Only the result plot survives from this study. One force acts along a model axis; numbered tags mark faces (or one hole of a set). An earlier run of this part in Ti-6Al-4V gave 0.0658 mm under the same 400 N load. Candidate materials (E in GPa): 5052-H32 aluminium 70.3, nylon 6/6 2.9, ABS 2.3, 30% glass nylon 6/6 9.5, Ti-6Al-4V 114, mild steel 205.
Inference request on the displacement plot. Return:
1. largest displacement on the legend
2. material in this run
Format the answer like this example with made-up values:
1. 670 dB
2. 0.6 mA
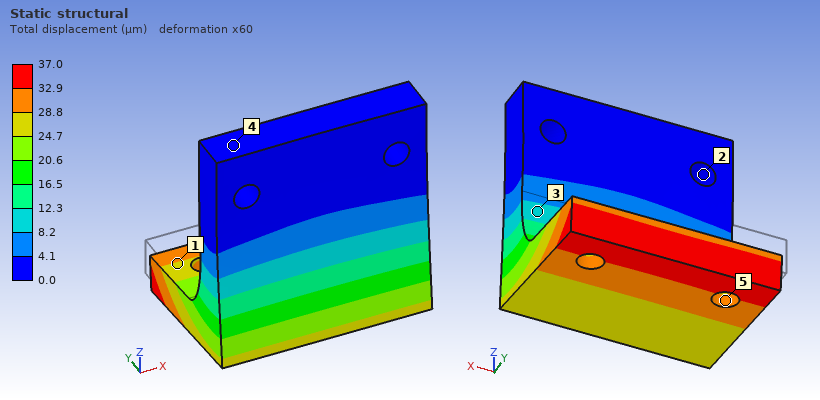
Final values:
1. 37.0 µm
2. mild steel
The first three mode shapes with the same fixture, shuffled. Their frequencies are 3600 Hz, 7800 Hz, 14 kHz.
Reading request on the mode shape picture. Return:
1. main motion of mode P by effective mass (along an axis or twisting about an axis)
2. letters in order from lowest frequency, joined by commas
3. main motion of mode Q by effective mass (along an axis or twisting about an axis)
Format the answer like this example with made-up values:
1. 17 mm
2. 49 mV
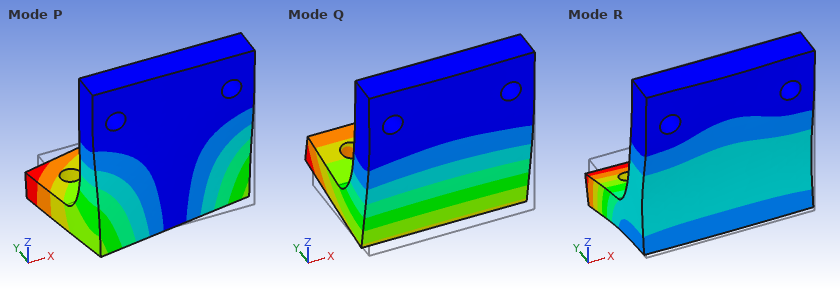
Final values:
1. along X
2. Q, P, R
3. along Y
